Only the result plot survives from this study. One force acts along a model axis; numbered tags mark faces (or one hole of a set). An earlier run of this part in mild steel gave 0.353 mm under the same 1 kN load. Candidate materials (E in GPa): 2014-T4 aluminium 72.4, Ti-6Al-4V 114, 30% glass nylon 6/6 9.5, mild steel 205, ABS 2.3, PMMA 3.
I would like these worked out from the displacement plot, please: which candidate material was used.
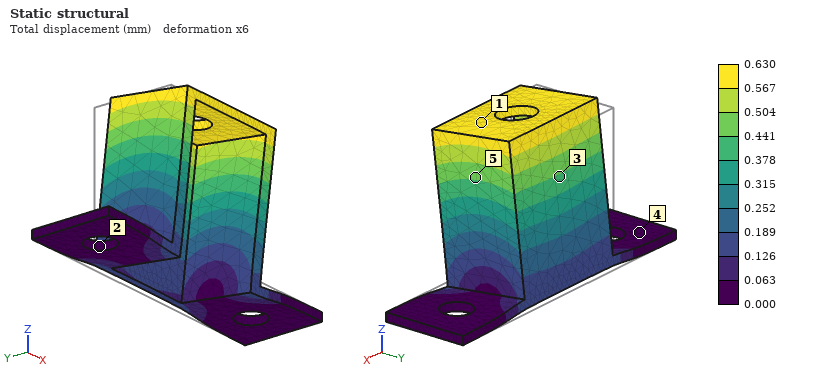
Ti-6Al-4V
